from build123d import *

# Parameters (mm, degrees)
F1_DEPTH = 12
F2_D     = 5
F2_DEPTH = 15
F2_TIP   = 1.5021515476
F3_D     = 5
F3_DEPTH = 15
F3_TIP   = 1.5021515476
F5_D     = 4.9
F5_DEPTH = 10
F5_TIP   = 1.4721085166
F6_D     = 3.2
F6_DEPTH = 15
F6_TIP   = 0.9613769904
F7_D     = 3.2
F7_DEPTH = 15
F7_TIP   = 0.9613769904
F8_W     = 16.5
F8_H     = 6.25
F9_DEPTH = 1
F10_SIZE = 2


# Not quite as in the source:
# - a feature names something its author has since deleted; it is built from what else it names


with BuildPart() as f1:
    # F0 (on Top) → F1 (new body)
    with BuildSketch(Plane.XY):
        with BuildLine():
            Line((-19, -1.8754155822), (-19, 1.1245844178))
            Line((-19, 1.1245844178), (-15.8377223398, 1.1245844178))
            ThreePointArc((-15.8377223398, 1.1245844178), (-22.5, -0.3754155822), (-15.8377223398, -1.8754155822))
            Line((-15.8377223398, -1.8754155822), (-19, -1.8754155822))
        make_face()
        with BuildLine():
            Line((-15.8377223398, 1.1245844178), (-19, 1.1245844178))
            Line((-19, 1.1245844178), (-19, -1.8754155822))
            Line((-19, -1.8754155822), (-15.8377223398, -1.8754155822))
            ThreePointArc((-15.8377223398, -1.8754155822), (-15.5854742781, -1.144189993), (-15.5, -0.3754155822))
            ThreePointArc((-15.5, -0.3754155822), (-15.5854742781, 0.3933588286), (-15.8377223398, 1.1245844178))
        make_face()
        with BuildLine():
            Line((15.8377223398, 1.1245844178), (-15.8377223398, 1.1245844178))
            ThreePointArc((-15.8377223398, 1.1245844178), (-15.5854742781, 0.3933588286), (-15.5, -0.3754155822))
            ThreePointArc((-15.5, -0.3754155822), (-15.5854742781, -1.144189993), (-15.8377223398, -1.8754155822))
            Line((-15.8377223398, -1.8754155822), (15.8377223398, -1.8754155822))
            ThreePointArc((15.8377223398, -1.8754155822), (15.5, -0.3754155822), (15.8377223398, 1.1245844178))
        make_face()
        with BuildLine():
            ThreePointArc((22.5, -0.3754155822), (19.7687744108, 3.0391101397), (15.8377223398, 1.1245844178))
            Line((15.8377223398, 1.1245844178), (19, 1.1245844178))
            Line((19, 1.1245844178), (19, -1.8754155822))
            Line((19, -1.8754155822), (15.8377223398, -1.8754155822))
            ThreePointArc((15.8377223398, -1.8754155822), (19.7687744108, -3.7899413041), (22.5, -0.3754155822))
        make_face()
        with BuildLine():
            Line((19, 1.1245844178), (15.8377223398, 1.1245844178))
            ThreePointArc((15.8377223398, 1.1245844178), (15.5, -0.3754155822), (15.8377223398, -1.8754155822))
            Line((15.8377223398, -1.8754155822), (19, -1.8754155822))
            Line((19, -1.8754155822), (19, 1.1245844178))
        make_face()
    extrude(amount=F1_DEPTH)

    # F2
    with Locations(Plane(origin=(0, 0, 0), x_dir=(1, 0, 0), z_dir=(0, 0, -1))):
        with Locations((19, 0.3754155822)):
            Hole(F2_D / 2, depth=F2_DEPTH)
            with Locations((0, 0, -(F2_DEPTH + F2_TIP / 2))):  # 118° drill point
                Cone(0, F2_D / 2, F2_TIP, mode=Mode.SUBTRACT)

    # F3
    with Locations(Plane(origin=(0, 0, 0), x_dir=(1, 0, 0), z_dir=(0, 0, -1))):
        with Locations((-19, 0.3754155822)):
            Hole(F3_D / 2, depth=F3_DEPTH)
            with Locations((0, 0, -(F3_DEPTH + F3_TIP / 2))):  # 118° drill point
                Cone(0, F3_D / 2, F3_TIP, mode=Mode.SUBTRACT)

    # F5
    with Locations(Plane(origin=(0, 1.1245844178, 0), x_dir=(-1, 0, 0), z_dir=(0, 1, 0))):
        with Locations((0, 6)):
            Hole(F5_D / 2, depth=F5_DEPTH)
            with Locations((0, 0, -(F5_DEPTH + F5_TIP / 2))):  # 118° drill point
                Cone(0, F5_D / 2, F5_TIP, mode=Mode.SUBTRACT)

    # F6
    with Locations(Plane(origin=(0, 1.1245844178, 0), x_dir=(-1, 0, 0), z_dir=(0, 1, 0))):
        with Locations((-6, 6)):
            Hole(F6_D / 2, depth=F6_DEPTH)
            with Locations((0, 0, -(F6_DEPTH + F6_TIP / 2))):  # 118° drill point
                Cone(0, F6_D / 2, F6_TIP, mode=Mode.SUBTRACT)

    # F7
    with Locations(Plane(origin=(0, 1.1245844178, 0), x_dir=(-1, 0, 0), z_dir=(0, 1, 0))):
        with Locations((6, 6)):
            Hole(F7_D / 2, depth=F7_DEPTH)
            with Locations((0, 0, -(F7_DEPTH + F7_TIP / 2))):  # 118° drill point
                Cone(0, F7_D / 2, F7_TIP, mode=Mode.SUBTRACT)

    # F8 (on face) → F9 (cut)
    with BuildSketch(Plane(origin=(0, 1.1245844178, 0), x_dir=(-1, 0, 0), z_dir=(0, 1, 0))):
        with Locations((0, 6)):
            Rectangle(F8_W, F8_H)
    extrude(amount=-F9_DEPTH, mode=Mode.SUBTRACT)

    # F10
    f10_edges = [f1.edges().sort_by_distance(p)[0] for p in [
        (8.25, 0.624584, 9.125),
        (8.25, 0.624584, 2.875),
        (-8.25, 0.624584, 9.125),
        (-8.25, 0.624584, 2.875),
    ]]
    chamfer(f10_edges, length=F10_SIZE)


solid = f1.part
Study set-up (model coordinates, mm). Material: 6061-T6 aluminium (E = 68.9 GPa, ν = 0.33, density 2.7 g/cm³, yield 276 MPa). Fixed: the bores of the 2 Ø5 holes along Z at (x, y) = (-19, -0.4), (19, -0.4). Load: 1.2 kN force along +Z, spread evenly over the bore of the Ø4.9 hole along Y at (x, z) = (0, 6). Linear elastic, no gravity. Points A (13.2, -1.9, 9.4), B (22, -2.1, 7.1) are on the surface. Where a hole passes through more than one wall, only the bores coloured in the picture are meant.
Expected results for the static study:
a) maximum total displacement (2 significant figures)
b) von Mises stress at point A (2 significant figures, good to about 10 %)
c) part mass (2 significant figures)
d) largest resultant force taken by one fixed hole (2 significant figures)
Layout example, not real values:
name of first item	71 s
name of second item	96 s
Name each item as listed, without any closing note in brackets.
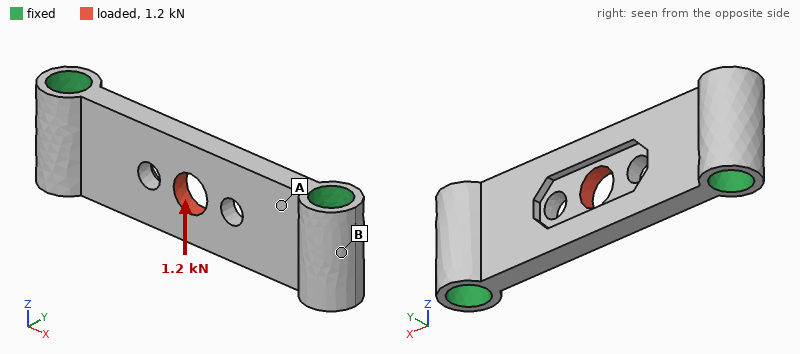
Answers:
maximum total displacement	28 µm
von Mises stress at point A	41 MPa
part mass	3.8 g
largest resultant force taken by one fixed hole	600 N
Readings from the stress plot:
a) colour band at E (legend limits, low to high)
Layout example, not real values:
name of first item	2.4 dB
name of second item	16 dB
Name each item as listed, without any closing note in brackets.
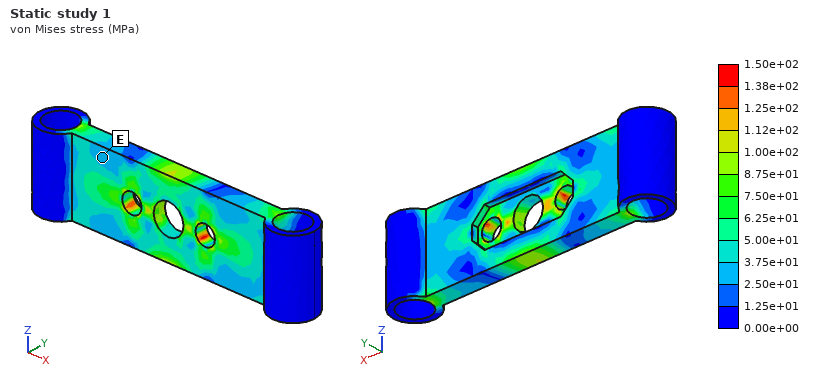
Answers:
colour band at E	2.50e+01 to 3.75e+01 MPa
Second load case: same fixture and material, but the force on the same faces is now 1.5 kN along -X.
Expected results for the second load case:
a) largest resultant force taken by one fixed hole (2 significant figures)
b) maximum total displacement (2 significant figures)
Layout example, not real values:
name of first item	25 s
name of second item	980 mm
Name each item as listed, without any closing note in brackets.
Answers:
largest resultant force taken by one fixed hole	750 N
maximum total displacement	8.8 µm
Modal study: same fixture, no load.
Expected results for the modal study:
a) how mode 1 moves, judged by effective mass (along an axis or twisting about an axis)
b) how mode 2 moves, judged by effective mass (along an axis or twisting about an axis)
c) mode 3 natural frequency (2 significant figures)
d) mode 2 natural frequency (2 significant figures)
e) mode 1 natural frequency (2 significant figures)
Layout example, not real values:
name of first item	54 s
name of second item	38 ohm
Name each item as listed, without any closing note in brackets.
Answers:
how mode 1 moves, judged by effective mass	along Y
how mode 2 moves, judged by effective mass	twisting about X
mode 3 natural frequency	35 kHz
mode 2 natural frequency	24 kHz
mode 1 natural frequency	15 kHz
